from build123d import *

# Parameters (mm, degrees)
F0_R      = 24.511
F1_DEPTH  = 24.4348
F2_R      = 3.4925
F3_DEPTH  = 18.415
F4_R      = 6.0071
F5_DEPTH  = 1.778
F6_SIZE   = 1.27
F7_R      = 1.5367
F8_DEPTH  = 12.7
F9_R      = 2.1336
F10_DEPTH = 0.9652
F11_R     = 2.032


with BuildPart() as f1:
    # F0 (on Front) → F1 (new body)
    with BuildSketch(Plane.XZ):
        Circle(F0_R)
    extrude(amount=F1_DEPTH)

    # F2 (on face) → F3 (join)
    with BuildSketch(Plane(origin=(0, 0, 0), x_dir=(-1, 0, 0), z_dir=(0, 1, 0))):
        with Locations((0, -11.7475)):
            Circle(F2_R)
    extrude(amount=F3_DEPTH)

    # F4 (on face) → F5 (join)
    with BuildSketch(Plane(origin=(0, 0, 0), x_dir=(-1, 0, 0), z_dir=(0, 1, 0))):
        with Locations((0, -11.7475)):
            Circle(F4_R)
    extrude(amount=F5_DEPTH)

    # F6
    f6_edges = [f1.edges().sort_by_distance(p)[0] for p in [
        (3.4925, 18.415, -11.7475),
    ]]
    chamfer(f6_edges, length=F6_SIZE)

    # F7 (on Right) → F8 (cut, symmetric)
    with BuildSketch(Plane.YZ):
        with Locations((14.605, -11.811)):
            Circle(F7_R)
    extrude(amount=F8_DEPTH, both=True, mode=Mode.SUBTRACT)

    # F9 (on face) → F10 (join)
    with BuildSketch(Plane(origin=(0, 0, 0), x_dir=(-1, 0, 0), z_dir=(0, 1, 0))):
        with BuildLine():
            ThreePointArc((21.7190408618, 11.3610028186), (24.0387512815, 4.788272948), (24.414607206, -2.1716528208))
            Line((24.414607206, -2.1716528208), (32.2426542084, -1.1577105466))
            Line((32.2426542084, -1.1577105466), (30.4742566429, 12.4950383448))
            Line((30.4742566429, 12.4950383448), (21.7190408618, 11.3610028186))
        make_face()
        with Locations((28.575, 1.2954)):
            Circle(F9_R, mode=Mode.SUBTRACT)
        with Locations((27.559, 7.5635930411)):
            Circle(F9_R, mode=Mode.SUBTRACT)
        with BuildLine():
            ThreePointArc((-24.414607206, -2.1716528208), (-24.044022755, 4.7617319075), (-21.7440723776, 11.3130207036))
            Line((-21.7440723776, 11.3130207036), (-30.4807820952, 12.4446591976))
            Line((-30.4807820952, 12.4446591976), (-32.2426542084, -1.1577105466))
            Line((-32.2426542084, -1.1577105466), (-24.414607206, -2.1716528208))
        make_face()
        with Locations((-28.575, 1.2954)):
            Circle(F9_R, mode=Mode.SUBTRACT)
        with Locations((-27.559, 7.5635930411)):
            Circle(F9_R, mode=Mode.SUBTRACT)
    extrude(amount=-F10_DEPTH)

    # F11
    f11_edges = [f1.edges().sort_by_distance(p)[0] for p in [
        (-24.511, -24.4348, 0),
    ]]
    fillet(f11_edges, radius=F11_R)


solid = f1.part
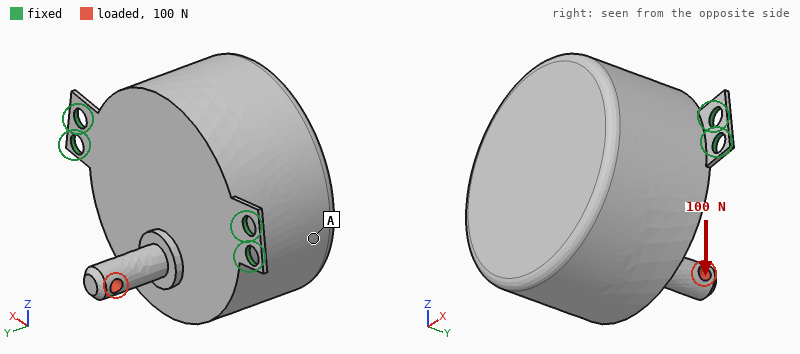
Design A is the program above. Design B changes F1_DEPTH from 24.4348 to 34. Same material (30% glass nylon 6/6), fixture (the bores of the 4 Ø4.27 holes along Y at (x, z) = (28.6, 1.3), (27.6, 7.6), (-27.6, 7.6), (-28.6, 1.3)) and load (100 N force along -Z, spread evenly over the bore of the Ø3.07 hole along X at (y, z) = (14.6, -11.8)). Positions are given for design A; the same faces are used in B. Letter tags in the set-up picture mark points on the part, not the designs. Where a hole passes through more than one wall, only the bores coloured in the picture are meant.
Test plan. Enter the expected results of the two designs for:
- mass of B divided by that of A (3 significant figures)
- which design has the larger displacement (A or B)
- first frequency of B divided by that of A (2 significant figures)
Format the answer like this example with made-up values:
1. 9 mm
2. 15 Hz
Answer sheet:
1. 1.38
2. B
3. 0.71
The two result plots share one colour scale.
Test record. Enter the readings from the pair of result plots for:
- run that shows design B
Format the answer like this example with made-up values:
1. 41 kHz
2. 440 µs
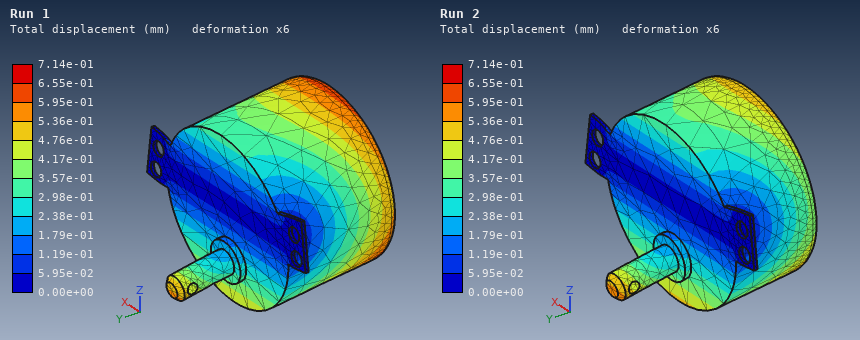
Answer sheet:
1. Run 1
